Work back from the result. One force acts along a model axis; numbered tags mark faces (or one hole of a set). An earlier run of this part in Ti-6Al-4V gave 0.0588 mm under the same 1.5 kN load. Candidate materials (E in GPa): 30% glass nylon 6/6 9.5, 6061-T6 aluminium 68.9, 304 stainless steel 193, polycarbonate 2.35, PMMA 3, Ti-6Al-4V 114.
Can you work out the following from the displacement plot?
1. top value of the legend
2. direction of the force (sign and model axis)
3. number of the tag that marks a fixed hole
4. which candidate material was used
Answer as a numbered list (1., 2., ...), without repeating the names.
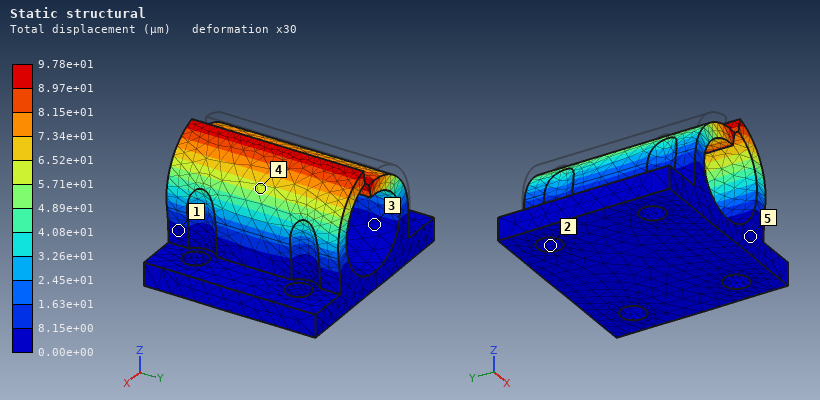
1. 9.78e+01 µm
2. +X
3. 2
4. 6061-T6 aluminium
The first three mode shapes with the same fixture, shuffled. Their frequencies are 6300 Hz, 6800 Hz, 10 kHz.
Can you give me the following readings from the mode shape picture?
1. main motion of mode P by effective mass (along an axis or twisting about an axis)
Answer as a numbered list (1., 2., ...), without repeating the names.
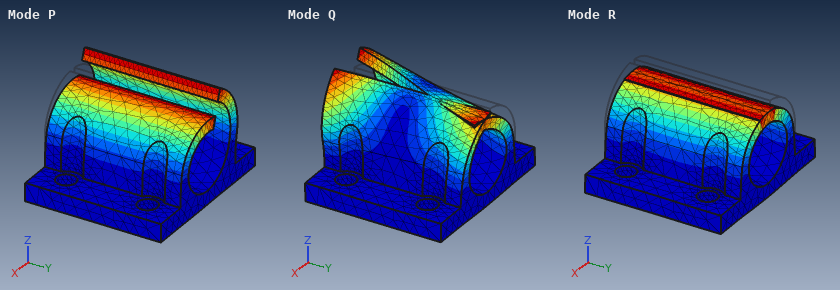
1. along X
